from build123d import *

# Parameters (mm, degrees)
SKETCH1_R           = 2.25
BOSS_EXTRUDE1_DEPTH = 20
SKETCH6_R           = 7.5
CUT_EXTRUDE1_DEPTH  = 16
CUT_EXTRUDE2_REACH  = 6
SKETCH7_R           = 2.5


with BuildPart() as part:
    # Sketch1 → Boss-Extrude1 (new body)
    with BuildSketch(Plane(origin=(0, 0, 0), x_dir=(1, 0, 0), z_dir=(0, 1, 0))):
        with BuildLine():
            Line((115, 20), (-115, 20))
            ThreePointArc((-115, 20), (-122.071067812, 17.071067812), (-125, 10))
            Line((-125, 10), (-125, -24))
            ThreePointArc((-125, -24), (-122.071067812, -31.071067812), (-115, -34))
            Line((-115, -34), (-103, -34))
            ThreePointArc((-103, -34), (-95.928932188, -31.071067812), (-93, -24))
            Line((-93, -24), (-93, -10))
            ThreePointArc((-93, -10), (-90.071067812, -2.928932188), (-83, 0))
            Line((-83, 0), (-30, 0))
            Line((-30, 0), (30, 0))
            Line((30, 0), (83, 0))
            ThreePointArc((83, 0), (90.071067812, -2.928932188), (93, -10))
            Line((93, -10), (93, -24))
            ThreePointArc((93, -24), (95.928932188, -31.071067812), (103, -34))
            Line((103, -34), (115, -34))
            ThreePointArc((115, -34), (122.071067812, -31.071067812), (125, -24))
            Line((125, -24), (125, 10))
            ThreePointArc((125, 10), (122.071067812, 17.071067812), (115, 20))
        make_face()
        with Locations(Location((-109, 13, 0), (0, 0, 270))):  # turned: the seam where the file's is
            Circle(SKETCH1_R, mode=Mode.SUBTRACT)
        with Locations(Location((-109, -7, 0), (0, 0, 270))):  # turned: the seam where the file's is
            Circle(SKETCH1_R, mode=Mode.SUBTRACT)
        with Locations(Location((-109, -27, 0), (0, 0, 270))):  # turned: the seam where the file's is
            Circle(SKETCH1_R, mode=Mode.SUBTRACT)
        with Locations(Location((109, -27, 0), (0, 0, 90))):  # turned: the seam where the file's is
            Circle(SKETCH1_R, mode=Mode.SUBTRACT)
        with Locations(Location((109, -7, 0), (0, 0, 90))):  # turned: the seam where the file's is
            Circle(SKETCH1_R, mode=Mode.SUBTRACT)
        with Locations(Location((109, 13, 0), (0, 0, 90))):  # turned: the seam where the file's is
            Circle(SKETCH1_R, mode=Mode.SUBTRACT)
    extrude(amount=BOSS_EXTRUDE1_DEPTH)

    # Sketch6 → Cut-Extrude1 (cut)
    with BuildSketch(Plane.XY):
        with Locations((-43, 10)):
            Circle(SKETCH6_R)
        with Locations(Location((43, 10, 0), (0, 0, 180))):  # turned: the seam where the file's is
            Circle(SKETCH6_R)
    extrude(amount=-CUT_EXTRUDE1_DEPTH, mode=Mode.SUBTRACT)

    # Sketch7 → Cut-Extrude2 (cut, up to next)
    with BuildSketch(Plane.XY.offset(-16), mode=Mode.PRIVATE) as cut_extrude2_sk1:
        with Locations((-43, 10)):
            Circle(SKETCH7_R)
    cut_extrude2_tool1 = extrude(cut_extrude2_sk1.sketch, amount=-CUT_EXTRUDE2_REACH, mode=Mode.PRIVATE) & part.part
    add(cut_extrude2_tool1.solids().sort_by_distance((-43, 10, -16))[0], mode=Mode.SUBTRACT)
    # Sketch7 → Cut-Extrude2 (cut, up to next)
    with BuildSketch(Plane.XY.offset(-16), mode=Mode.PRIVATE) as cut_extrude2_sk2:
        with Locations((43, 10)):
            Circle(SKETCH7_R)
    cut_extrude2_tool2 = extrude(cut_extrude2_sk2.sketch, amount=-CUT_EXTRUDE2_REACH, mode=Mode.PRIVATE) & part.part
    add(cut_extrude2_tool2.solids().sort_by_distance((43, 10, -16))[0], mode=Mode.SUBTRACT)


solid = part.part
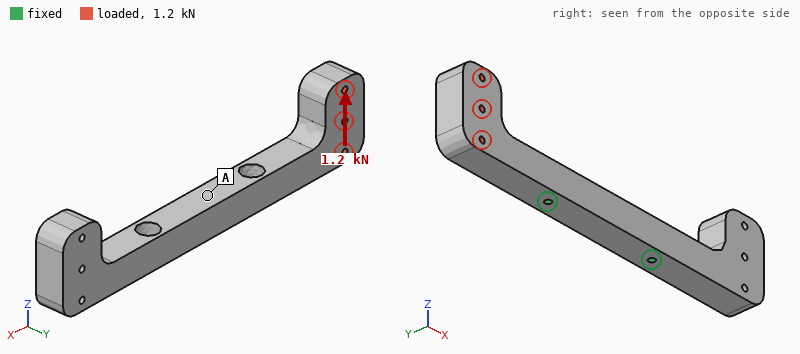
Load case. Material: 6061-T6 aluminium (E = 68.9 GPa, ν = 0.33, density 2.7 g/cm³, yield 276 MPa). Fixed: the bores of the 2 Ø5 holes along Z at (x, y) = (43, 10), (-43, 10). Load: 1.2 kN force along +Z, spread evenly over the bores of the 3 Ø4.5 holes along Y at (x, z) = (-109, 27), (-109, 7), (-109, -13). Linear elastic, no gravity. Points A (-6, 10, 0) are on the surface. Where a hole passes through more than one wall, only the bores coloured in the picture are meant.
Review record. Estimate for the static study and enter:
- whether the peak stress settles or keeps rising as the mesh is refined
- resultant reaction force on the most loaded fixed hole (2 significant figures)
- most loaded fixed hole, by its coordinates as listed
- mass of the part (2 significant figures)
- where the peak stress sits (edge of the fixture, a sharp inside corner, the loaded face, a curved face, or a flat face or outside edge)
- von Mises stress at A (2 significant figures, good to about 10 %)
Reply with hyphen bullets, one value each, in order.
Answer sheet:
- keeps rising
- 3.2 kN
- (-43, 10)
- 360 g
- edge of the fixture
- 21 MPa
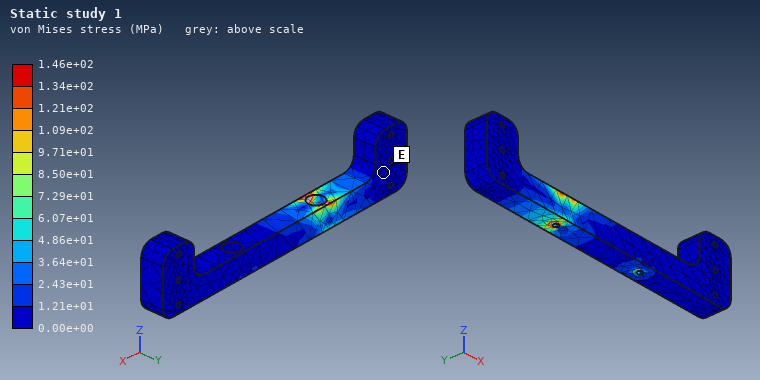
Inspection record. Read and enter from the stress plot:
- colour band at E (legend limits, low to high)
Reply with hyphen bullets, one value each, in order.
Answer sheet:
- 0.00e+00 to 1.21e+01 MPa
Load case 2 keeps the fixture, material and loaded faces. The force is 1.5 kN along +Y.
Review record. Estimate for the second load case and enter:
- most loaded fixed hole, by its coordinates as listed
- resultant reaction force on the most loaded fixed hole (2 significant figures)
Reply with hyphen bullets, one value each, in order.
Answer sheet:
- (-43, 10)
- 2.4 kN
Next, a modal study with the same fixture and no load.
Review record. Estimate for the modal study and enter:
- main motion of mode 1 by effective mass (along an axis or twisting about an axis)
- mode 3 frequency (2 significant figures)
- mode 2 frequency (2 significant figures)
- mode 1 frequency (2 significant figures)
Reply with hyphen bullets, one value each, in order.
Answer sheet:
- along Y
- 900 Hz
- 900 Hz
- 760 Hz
